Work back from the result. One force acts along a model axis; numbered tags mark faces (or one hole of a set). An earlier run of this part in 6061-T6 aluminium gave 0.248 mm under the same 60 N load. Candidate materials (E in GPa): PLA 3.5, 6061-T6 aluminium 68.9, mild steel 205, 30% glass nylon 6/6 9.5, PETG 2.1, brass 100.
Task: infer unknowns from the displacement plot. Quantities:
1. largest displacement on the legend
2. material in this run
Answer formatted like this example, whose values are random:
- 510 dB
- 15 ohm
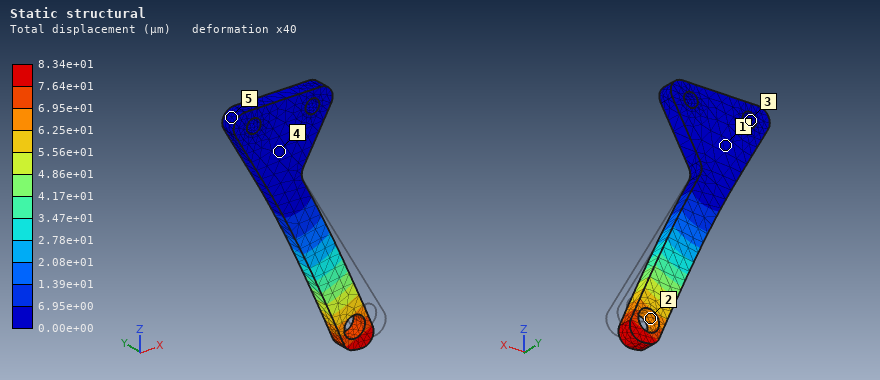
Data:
- 8.34e+01 µm
- mild steel
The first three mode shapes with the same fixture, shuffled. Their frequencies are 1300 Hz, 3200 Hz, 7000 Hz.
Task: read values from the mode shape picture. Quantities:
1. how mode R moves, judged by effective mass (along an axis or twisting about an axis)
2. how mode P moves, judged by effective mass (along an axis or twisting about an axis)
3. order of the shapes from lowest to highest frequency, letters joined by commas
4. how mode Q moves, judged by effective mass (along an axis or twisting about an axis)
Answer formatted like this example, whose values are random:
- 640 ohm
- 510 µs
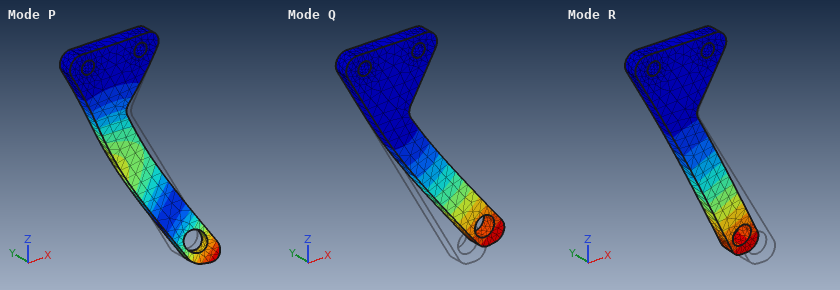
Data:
- along Y
- along Y
- R, Q, P
- along X
